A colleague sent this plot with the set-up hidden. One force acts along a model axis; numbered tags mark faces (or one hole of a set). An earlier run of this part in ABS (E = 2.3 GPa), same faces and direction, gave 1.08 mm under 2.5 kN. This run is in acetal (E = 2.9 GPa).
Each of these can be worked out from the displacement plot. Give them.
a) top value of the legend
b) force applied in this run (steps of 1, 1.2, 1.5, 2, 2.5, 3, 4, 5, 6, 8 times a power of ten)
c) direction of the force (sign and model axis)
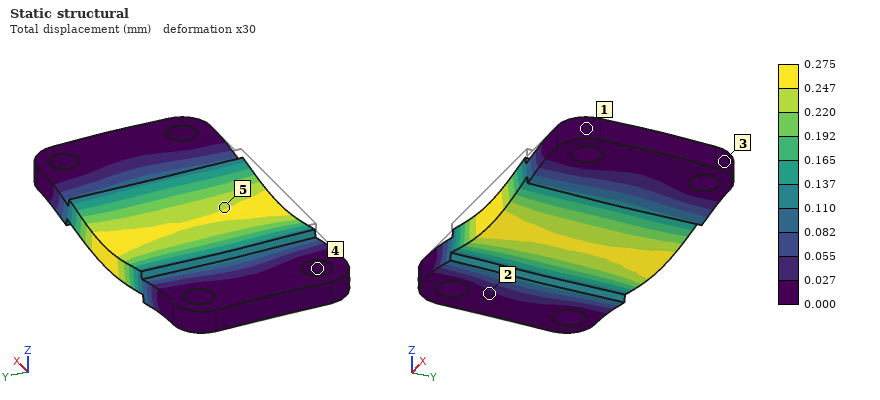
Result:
0.275 mm
800 N
-Z
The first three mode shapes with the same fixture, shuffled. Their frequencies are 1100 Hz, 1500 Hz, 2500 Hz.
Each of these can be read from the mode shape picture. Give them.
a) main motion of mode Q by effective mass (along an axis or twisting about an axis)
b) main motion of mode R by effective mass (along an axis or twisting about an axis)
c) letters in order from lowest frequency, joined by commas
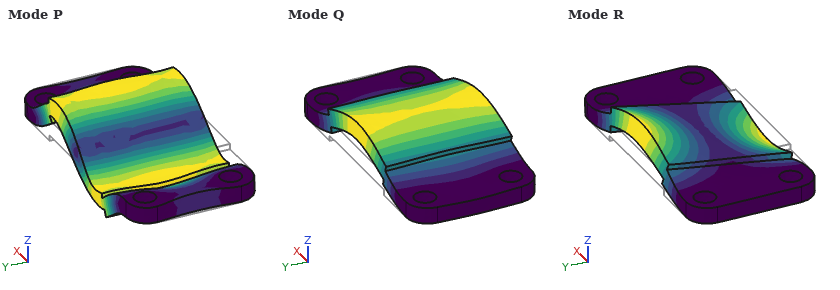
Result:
along Z
twisting about X
Q, R, P
